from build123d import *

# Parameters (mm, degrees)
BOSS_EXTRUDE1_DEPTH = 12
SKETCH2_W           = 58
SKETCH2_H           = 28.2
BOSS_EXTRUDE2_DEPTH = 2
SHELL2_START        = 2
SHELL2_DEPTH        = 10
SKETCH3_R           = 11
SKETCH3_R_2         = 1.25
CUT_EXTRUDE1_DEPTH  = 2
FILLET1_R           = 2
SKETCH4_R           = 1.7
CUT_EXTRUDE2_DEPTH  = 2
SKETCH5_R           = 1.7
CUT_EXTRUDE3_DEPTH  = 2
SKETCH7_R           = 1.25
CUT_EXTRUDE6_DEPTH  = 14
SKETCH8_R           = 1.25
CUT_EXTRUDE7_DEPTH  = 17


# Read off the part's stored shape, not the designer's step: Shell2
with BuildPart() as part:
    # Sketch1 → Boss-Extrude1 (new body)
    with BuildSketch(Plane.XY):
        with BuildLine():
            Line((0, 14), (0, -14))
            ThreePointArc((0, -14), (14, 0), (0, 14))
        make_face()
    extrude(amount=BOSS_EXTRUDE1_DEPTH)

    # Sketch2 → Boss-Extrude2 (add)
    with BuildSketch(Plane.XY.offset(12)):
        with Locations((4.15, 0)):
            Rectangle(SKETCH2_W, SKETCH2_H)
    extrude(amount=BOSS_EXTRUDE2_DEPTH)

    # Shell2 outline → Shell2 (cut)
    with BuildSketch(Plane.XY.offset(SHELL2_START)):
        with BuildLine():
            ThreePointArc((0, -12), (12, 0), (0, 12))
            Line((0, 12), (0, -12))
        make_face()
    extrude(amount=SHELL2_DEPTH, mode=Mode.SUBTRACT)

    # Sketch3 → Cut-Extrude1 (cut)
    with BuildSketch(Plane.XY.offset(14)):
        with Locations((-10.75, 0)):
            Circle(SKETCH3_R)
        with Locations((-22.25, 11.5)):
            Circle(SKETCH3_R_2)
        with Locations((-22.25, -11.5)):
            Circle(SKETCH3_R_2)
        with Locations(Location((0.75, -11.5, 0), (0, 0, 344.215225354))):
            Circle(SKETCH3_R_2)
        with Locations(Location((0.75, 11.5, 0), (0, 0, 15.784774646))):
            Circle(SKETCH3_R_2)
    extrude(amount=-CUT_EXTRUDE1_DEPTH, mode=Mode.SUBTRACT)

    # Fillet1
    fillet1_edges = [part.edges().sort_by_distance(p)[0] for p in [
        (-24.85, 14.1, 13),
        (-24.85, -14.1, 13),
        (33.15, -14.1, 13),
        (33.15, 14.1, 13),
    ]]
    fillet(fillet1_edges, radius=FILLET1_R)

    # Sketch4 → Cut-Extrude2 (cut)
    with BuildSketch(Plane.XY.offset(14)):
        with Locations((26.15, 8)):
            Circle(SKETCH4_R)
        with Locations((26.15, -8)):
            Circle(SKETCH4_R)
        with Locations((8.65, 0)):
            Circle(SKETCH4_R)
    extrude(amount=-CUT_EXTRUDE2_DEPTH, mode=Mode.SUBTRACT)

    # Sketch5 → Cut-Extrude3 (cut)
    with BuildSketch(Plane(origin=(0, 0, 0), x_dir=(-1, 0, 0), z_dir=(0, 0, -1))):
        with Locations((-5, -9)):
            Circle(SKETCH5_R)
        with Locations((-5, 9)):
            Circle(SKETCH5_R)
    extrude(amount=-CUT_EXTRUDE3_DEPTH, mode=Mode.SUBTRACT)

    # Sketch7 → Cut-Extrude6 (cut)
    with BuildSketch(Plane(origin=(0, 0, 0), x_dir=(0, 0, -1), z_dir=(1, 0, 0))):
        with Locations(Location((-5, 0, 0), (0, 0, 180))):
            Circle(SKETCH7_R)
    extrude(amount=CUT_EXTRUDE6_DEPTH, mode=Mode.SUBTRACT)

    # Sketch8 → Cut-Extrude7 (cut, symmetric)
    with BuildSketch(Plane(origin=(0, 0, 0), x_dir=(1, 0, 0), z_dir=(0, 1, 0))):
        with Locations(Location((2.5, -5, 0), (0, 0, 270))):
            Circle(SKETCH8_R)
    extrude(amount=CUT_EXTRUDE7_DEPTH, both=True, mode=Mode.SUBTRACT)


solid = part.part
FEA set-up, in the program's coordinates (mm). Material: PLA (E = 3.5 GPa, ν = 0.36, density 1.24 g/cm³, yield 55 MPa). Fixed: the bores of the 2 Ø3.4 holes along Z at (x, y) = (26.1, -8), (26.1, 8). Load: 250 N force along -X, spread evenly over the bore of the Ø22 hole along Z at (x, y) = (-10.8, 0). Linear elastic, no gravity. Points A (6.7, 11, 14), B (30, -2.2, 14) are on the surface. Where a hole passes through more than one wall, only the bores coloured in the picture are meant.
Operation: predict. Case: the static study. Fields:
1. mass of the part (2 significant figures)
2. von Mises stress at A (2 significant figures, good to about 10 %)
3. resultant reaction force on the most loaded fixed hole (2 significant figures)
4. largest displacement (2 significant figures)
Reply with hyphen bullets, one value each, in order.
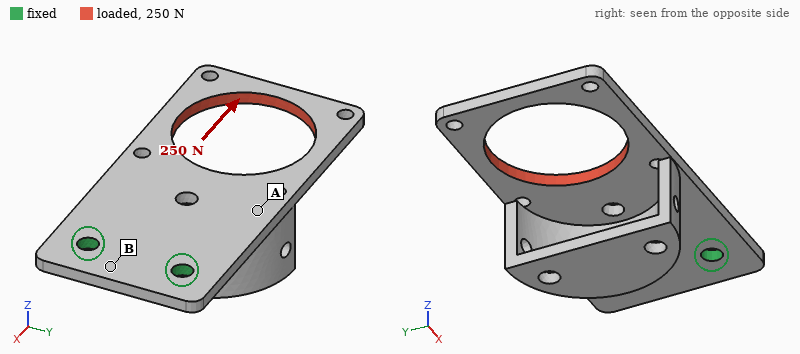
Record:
- 4.7 g
- 7.0 MPa
- 130 N
- 0.34 mm
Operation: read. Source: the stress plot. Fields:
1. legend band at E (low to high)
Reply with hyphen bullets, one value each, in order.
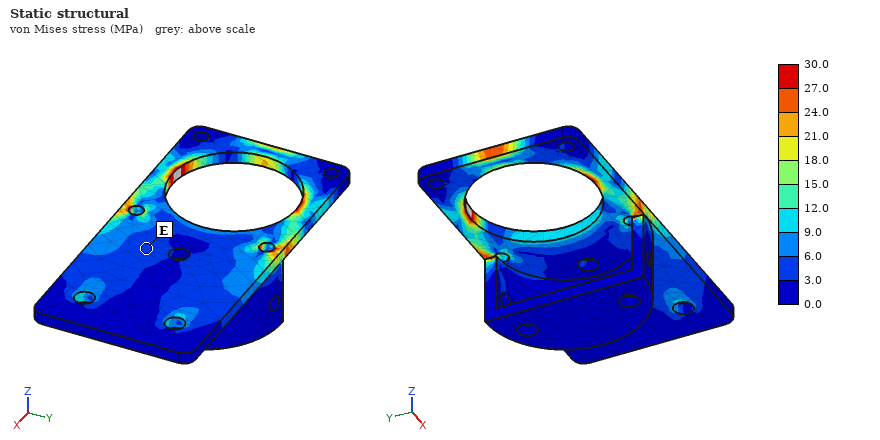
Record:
- 3.0 to 6.0 MPa
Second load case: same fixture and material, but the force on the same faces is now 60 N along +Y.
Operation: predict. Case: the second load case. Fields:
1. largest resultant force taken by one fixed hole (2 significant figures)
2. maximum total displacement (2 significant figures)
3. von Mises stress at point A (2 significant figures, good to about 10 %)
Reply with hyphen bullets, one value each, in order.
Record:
- 130 N
- 0.45 mm
- 3.1 MPa
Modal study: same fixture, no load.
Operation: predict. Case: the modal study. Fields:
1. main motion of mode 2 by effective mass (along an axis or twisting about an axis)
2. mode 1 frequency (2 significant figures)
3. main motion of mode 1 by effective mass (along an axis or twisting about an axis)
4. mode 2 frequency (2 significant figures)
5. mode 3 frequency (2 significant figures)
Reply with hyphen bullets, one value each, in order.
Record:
- along Z
- 270 Hz
- along Z
- 820 Hz
- 910 Hz
